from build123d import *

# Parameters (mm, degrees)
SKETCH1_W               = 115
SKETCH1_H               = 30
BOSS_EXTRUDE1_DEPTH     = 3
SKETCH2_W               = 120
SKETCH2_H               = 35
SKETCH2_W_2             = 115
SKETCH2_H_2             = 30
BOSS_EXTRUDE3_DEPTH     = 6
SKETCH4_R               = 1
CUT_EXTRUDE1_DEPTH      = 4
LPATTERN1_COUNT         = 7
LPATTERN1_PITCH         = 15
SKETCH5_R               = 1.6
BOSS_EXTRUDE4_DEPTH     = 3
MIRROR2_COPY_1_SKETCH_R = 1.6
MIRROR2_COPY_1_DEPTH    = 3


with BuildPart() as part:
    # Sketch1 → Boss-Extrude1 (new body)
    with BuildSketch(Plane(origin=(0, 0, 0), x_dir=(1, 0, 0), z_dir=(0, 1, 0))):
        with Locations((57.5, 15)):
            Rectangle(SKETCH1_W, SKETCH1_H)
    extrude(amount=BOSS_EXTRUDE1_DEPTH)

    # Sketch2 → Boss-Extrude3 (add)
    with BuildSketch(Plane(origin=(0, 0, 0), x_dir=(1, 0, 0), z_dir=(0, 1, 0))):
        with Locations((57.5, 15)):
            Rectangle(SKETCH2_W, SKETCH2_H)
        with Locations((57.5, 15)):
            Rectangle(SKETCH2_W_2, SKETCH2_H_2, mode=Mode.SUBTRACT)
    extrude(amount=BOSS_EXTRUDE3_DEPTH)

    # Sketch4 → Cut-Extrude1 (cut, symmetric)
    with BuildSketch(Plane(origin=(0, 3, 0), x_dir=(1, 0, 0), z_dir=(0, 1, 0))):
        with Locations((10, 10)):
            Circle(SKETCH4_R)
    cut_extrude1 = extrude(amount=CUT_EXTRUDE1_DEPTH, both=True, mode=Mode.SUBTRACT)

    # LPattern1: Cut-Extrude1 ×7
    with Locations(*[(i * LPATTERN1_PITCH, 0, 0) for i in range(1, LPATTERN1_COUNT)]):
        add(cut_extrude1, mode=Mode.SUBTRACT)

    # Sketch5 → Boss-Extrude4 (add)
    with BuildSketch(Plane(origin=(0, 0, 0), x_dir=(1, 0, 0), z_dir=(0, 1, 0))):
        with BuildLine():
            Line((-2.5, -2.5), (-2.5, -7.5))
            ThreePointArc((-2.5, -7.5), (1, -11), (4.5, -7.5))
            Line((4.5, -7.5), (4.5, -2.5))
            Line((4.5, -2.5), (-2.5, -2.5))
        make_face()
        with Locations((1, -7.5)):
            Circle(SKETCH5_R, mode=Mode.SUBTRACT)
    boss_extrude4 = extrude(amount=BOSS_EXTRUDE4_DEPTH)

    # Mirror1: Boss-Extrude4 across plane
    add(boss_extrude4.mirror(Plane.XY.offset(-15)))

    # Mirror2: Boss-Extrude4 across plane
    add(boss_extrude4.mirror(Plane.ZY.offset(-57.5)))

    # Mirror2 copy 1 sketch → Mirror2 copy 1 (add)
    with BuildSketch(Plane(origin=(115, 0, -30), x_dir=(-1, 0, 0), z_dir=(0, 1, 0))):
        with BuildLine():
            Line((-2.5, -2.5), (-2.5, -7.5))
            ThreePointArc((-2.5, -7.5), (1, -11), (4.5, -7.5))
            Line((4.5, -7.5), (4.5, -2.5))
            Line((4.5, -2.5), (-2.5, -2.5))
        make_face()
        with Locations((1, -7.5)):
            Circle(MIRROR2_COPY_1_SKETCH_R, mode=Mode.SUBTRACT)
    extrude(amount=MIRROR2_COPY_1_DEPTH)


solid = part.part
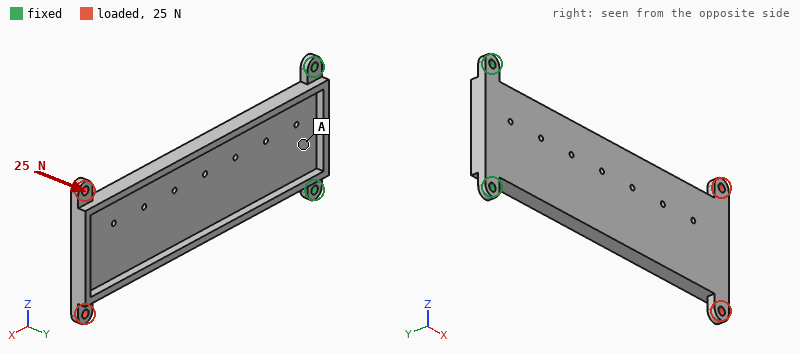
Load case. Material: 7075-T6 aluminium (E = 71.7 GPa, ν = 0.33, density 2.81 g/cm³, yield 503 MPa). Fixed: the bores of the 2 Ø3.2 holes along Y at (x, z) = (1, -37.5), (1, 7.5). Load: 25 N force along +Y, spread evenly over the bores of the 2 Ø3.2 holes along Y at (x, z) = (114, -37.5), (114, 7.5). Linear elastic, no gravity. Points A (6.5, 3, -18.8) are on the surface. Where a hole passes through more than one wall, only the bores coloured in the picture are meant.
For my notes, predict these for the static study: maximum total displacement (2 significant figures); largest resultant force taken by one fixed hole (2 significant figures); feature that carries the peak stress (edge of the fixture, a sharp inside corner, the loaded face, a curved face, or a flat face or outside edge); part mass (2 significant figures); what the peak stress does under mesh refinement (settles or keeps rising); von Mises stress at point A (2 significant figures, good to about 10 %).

1.4 mm
62 N
edge of the fixture
43 g
keeps rising
15 MPa
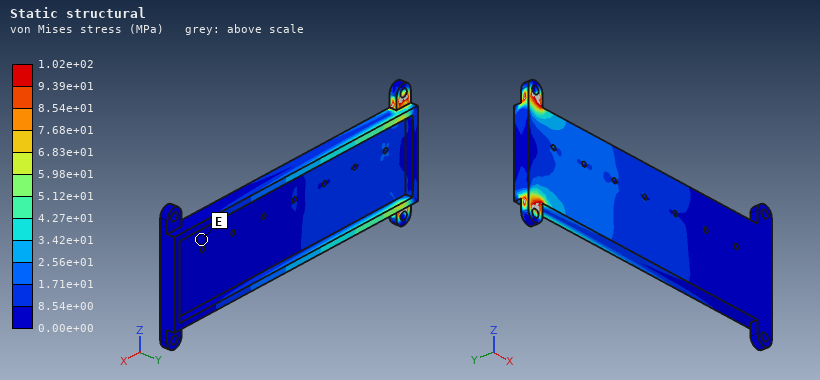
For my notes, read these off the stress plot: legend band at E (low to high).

0.00e+00 to 8.54e+00 MPa
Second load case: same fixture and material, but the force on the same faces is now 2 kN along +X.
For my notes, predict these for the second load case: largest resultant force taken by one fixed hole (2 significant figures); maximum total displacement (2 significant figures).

1.1 kN
0.51 mm
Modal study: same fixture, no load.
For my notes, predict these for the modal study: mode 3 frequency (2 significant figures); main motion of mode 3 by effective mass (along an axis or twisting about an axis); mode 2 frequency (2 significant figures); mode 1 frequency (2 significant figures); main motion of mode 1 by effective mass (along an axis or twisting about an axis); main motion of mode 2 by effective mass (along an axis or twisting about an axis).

1300 Hz
along Y
1000 Hz
190 Hz
along Y
twisting about X
